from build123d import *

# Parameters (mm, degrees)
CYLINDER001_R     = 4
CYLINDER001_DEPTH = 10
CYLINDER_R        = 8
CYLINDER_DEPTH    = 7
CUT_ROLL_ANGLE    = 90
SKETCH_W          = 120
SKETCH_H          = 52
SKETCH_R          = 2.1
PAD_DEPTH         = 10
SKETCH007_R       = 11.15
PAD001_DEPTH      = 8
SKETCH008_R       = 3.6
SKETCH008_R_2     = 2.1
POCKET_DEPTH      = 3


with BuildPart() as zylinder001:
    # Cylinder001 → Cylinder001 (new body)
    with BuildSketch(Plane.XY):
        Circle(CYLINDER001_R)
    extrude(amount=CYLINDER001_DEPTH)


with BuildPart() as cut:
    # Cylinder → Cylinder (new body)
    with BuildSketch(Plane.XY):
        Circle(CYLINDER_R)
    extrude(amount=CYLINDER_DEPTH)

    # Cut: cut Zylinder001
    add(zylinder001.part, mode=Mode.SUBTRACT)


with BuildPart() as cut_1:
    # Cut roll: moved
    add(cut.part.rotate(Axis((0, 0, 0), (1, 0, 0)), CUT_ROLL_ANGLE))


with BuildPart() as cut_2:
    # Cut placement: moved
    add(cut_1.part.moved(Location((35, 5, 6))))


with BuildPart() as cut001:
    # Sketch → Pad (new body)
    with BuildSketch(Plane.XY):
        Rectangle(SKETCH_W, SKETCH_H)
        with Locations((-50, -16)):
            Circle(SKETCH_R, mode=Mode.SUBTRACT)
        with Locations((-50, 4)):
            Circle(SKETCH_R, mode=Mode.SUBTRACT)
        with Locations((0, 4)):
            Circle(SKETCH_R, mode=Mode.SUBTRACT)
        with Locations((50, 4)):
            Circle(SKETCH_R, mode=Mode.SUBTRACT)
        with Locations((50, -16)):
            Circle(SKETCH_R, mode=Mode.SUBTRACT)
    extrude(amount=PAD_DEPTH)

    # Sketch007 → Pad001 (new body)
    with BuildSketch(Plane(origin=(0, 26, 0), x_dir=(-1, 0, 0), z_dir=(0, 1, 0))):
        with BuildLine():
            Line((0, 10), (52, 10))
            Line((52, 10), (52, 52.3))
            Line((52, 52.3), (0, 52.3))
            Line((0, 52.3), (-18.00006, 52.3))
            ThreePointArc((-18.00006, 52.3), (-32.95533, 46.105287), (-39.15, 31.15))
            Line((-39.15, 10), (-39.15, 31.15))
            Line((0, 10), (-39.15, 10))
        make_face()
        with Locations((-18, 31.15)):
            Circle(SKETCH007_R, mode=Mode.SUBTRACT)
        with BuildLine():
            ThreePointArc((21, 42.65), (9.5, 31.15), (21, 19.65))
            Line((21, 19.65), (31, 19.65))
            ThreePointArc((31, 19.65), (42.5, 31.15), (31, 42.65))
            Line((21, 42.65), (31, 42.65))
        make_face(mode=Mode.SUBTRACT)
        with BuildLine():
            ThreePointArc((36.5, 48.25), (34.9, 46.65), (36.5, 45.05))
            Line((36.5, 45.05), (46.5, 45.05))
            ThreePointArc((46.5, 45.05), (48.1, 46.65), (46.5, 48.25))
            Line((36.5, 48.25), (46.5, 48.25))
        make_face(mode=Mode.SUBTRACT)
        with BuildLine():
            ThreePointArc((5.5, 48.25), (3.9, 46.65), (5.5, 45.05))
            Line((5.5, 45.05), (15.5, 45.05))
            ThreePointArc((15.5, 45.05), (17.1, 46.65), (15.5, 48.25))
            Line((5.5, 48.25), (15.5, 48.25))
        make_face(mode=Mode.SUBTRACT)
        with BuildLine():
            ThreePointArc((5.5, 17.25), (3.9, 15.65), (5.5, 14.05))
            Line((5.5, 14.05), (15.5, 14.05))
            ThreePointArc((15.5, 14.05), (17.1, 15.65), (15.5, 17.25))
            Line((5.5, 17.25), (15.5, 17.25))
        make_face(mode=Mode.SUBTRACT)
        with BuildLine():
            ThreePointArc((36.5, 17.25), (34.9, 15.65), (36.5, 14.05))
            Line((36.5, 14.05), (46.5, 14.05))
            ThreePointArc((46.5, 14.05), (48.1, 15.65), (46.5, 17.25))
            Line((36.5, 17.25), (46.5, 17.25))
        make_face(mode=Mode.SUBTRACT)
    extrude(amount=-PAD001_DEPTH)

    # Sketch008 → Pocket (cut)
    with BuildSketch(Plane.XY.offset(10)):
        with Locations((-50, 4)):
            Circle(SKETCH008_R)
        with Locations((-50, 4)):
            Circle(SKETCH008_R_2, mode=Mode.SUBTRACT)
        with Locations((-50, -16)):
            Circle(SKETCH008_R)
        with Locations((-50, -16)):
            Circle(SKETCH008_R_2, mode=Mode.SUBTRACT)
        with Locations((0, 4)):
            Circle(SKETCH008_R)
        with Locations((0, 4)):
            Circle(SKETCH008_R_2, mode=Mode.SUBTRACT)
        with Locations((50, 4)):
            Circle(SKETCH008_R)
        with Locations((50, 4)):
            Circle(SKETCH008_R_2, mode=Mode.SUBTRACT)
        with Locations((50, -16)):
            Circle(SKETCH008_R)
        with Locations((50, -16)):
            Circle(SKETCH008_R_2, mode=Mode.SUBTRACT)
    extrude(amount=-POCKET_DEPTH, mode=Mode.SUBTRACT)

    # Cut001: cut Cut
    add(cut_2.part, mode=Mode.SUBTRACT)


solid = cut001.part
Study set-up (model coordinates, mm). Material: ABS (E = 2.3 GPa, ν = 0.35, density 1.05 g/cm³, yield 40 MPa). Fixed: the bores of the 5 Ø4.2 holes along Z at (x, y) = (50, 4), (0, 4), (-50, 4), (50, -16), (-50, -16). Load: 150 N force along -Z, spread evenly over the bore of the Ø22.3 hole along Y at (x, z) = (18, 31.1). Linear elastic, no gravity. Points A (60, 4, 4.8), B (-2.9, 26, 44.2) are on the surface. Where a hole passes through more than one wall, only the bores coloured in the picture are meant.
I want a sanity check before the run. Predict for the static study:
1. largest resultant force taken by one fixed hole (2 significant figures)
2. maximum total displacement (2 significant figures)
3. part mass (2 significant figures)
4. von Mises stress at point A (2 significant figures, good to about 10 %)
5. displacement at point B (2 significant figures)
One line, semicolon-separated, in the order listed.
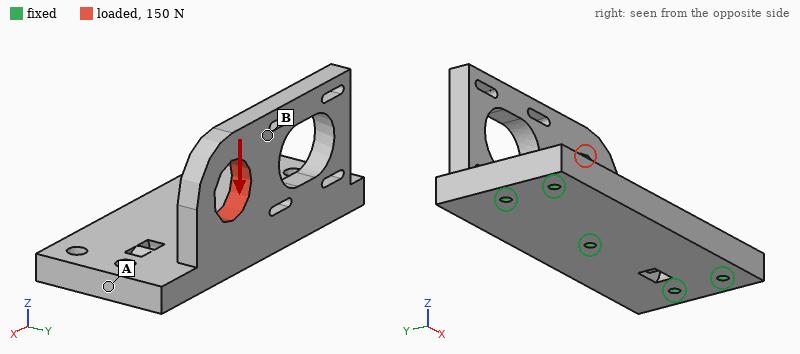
98 N; 0.17 mm; 85 g; 0.86 MPa; 0.12 mm
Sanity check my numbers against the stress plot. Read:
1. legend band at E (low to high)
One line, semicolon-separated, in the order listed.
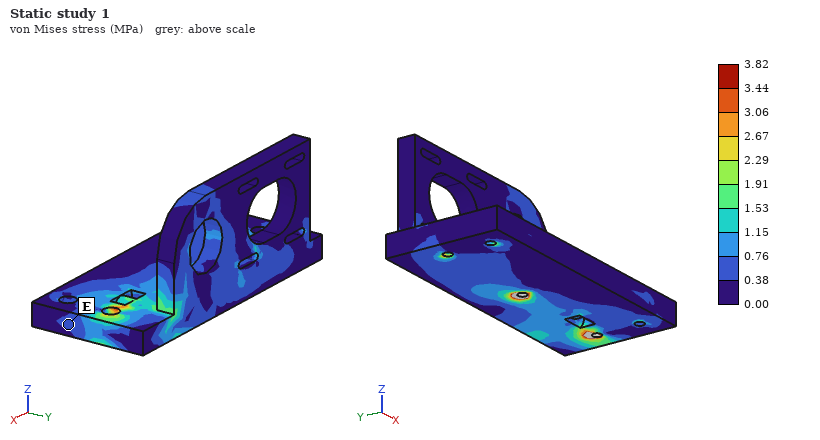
0.38 to 0.76 MPa
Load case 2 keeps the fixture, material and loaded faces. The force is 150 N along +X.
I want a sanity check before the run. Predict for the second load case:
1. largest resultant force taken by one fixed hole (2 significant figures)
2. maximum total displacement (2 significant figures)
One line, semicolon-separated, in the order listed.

73 N; 72 µm
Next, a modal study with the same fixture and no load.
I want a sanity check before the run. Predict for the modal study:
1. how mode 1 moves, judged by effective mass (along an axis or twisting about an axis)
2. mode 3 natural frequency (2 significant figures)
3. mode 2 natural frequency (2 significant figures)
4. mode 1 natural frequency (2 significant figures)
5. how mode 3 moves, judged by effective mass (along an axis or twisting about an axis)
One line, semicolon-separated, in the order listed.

along Y; 1700 Hz; 1100 Hz; 610 Hz; along Z
